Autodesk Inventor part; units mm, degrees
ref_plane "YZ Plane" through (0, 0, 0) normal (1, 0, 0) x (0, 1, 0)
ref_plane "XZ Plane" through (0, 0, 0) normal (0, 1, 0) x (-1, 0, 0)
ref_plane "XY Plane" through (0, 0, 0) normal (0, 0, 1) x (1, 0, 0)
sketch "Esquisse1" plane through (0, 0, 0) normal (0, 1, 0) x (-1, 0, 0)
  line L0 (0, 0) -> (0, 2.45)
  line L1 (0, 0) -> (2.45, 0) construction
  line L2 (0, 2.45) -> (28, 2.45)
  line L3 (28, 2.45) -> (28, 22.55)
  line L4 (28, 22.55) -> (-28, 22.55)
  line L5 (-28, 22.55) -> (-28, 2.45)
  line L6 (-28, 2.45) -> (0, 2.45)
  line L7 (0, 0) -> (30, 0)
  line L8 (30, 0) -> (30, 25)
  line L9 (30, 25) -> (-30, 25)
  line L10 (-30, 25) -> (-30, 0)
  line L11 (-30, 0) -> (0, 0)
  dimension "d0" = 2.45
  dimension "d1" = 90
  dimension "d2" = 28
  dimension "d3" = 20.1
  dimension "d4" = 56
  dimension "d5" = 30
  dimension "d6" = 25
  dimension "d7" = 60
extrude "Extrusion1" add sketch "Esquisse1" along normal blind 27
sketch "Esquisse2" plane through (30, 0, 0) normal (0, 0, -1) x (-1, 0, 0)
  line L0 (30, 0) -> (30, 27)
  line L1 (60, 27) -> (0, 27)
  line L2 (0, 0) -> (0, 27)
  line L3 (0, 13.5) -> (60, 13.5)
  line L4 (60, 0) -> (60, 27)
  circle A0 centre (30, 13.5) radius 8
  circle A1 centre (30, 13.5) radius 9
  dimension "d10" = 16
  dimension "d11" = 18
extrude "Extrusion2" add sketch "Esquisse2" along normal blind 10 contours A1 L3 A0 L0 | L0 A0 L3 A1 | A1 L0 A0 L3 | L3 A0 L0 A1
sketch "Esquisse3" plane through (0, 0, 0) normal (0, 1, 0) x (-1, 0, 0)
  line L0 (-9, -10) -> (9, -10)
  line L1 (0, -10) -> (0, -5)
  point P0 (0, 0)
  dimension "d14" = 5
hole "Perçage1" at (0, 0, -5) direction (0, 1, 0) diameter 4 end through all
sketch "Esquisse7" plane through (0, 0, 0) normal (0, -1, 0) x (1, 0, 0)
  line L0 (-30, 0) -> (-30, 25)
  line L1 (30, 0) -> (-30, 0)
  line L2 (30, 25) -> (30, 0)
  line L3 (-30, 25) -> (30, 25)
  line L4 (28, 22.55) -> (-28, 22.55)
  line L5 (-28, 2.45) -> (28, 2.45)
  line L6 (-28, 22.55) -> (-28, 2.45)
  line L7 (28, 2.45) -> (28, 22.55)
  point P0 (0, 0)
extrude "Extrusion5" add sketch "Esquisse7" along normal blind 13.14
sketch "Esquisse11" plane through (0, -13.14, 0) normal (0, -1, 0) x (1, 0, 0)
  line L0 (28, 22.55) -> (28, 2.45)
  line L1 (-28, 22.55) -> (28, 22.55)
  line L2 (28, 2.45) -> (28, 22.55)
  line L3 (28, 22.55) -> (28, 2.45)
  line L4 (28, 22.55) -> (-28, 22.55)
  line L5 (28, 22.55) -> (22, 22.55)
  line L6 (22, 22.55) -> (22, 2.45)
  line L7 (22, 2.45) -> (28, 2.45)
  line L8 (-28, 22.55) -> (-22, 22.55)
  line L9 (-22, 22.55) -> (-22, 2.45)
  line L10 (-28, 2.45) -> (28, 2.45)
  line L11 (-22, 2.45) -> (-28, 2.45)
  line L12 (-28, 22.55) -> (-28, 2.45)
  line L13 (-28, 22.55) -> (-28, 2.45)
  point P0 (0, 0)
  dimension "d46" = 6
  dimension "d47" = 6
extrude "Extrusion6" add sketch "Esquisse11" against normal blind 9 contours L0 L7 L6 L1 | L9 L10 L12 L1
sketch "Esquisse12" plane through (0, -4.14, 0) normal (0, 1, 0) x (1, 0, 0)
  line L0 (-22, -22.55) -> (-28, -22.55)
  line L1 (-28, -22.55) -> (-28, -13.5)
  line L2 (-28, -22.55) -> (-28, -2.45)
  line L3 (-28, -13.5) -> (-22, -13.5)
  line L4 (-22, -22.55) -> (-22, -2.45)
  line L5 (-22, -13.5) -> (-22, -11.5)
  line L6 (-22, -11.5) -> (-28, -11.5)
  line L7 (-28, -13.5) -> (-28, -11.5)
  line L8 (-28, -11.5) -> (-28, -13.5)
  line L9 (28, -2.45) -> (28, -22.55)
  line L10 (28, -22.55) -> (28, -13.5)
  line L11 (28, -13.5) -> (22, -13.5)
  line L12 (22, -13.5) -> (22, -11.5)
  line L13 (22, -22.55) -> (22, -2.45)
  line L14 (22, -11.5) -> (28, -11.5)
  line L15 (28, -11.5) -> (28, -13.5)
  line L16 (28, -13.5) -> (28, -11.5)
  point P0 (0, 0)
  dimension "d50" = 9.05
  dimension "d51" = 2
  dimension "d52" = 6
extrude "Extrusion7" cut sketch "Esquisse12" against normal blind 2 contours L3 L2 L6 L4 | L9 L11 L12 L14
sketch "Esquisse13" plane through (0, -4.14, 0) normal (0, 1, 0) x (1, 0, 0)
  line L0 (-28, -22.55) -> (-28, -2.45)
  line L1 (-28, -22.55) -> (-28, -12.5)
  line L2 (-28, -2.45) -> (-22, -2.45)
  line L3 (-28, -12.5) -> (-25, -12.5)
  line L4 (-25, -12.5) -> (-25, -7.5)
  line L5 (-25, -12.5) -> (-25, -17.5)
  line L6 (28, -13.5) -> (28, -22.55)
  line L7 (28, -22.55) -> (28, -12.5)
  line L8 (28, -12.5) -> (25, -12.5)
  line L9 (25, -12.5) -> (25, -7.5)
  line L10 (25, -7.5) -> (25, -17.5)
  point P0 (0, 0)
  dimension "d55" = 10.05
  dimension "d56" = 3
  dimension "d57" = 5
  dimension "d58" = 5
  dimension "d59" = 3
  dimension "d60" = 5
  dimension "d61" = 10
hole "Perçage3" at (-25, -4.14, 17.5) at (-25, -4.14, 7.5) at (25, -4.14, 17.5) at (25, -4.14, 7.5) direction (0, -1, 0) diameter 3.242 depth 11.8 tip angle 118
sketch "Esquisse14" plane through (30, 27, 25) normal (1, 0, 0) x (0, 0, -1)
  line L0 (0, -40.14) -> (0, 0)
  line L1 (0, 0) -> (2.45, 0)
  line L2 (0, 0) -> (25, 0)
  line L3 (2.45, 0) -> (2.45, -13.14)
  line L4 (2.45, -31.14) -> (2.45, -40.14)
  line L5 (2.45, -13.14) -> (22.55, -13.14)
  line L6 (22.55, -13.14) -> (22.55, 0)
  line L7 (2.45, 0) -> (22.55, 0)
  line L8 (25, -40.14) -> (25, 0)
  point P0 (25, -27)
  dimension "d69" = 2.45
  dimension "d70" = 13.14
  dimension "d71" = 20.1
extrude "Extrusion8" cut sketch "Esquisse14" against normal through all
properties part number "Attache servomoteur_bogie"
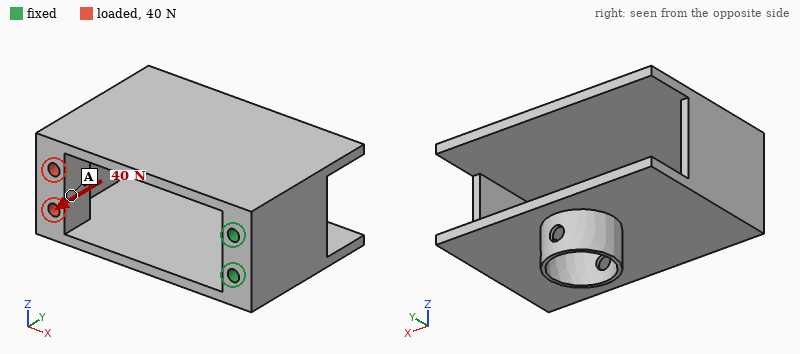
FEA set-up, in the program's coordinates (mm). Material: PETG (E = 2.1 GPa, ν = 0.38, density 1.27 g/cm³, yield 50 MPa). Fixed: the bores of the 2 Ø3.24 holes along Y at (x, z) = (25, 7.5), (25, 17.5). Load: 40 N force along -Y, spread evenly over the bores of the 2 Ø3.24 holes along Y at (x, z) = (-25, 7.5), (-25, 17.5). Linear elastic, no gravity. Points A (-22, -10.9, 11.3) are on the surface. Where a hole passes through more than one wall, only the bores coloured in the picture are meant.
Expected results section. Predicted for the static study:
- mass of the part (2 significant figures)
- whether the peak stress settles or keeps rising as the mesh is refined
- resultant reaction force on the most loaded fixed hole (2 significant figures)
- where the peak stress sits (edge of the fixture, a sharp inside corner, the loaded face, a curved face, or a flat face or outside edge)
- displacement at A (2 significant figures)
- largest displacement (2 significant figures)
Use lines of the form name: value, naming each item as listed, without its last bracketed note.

mass of the part: 21 g
whether the peak stress settles or keeps rising as the mesh is refined: keeps rising
resultant reaction force on the most loaded fixed hole: 20 N
where the peak stress sits: edge of the fixture
displacement at A: 0.65 mm
largest displacement: 0.87 mm
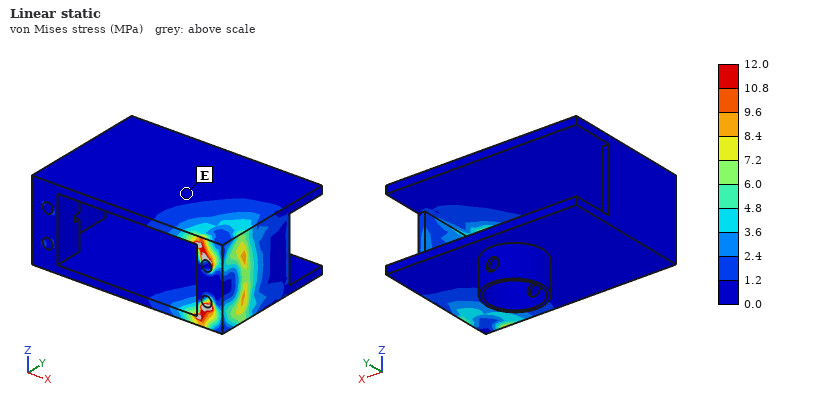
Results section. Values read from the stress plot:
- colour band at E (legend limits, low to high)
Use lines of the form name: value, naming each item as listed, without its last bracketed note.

colour band at E: 0.0 to 1.2 MPa
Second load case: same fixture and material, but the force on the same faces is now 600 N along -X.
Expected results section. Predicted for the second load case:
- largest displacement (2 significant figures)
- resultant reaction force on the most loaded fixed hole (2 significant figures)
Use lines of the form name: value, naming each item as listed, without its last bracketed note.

largest displacement: 0.66 mm
resultant reaction force on the most loaded fixed hole: 330 N
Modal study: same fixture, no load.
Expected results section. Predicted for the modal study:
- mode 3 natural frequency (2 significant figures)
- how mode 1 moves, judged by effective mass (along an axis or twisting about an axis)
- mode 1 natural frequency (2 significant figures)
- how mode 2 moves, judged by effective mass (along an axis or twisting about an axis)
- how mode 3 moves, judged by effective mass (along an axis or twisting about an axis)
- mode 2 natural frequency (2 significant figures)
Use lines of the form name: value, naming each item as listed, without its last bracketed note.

mode 3 natural frequency: 470 Hz
how mode 1 moves, judged by effective mass: along Z
mode 1 natural frequency: 200 Hz
how mode 2 moves, judged by effective mass: along Y
how mode 3 moves, judged by effective mass: twisting about X
mode 2 natural frequency: 370 Hz
